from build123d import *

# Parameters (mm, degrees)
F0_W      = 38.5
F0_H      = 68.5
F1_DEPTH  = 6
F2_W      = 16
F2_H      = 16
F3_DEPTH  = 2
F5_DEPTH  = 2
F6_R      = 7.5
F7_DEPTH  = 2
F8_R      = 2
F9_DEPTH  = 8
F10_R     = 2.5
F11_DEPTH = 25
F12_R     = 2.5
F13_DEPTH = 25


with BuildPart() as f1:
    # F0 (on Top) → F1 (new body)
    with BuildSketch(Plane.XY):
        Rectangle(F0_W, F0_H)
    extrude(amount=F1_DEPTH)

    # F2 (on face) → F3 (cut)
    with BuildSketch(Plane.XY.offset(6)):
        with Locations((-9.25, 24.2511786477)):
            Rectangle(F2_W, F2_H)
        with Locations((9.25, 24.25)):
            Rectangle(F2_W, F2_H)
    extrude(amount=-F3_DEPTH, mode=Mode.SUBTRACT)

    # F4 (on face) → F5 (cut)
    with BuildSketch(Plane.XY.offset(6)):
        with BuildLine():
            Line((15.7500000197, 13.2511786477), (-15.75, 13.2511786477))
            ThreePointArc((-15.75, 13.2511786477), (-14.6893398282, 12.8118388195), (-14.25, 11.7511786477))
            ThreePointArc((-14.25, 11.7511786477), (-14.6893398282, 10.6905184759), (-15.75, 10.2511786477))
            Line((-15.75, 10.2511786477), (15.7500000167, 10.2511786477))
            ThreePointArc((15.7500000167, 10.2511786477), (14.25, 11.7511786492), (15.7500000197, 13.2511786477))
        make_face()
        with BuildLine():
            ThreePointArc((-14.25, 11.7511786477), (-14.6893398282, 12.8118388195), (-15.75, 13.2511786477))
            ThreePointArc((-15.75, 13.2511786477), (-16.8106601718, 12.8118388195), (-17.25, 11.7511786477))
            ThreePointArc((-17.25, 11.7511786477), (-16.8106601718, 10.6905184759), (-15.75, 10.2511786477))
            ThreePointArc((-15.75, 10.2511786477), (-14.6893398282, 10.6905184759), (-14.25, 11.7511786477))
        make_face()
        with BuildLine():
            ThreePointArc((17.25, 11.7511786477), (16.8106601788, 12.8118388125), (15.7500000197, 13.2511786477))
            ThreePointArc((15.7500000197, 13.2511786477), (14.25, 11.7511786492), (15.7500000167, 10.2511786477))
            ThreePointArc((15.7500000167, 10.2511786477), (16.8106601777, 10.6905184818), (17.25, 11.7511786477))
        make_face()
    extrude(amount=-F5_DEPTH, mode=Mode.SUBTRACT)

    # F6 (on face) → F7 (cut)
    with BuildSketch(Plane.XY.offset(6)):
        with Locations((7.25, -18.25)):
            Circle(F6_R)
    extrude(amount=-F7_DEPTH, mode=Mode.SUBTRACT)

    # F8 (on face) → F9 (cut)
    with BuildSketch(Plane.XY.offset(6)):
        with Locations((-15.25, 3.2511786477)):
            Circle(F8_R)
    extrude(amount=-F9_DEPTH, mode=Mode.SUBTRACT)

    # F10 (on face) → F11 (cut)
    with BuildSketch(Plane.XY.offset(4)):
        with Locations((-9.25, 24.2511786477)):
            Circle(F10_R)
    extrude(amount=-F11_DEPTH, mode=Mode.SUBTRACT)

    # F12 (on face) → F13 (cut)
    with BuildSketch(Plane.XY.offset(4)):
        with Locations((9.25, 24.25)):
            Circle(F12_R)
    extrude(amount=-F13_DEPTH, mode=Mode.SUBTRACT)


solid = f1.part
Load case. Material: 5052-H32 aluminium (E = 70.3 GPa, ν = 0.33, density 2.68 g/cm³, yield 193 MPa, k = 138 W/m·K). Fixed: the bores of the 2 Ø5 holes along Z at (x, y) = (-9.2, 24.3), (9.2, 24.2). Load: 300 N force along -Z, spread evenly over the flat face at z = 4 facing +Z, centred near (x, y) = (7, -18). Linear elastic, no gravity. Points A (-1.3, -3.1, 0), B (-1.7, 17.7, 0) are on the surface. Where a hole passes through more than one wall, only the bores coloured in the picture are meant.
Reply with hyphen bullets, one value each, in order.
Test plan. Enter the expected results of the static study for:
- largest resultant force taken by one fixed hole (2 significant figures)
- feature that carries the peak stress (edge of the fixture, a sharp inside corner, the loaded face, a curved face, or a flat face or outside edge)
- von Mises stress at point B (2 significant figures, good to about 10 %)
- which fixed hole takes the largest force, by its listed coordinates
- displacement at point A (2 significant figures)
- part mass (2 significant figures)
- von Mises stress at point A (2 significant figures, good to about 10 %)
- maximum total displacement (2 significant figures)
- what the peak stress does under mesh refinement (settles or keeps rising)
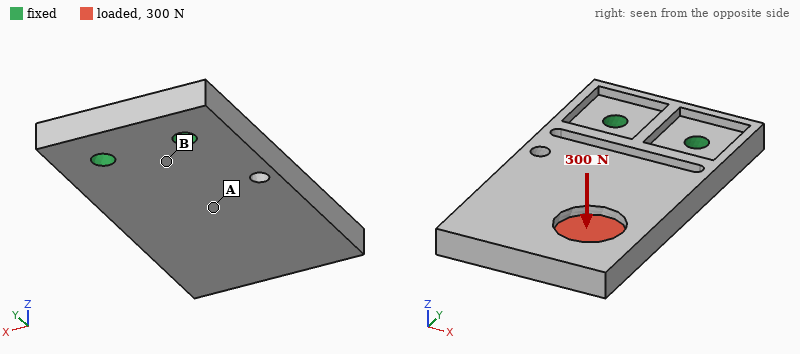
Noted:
- 250 N
- edge of the fixture
- 67 MPa
- (9.2, 24.2)
- 0.17 mm
- 38 g
- 23 MPa
- 0.50 mm
- keeps rising
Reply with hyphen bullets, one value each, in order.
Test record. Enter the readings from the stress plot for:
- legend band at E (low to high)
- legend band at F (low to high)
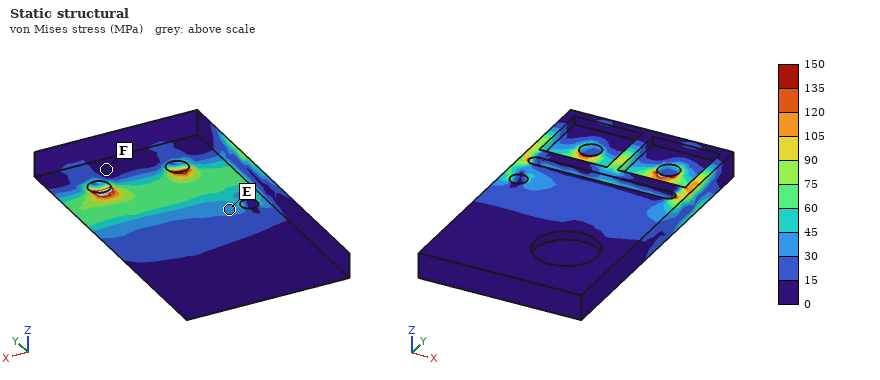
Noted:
- 30 to 45 MPa
- 0 to 15 MPa
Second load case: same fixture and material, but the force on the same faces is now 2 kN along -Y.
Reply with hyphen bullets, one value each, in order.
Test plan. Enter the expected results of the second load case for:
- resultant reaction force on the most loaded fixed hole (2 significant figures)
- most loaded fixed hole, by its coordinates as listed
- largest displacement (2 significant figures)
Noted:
- 1.7 kN
- (9.2, 24.2)
- 0.19 mm
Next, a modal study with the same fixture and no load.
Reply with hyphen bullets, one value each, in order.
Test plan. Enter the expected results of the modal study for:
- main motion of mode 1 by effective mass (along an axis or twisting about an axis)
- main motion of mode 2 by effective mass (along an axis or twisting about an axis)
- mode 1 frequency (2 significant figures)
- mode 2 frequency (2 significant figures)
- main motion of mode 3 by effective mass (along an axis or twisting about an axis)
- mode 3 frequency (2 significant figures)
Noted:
- along Z
- twisting about Y
- 1100 Hz
- 3800 Hz
- along X
- 5700 Hz
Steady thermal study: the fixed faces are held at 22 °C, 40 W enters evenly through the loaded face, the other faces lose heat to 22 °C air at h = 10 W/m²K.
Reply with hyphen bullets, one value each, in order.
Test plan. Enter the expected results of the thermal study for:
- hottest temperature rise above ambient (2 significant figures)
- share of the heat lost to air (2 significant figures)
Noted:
- 70 K
- 5.6 %
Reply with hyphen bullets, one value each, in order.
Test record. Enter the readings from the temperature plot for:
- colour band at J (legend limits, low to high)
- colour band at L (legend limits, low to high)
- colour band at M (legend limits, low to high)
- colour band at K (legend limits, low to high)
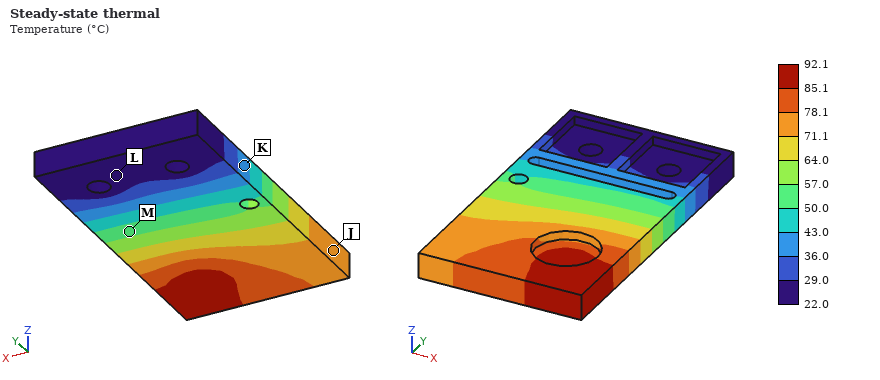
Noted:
- 71.1 to 78.1 °C
- 22.0 to 29.0 °C
- 50.0 to 57.0 °C
- 36.0 to 43.0 °C
